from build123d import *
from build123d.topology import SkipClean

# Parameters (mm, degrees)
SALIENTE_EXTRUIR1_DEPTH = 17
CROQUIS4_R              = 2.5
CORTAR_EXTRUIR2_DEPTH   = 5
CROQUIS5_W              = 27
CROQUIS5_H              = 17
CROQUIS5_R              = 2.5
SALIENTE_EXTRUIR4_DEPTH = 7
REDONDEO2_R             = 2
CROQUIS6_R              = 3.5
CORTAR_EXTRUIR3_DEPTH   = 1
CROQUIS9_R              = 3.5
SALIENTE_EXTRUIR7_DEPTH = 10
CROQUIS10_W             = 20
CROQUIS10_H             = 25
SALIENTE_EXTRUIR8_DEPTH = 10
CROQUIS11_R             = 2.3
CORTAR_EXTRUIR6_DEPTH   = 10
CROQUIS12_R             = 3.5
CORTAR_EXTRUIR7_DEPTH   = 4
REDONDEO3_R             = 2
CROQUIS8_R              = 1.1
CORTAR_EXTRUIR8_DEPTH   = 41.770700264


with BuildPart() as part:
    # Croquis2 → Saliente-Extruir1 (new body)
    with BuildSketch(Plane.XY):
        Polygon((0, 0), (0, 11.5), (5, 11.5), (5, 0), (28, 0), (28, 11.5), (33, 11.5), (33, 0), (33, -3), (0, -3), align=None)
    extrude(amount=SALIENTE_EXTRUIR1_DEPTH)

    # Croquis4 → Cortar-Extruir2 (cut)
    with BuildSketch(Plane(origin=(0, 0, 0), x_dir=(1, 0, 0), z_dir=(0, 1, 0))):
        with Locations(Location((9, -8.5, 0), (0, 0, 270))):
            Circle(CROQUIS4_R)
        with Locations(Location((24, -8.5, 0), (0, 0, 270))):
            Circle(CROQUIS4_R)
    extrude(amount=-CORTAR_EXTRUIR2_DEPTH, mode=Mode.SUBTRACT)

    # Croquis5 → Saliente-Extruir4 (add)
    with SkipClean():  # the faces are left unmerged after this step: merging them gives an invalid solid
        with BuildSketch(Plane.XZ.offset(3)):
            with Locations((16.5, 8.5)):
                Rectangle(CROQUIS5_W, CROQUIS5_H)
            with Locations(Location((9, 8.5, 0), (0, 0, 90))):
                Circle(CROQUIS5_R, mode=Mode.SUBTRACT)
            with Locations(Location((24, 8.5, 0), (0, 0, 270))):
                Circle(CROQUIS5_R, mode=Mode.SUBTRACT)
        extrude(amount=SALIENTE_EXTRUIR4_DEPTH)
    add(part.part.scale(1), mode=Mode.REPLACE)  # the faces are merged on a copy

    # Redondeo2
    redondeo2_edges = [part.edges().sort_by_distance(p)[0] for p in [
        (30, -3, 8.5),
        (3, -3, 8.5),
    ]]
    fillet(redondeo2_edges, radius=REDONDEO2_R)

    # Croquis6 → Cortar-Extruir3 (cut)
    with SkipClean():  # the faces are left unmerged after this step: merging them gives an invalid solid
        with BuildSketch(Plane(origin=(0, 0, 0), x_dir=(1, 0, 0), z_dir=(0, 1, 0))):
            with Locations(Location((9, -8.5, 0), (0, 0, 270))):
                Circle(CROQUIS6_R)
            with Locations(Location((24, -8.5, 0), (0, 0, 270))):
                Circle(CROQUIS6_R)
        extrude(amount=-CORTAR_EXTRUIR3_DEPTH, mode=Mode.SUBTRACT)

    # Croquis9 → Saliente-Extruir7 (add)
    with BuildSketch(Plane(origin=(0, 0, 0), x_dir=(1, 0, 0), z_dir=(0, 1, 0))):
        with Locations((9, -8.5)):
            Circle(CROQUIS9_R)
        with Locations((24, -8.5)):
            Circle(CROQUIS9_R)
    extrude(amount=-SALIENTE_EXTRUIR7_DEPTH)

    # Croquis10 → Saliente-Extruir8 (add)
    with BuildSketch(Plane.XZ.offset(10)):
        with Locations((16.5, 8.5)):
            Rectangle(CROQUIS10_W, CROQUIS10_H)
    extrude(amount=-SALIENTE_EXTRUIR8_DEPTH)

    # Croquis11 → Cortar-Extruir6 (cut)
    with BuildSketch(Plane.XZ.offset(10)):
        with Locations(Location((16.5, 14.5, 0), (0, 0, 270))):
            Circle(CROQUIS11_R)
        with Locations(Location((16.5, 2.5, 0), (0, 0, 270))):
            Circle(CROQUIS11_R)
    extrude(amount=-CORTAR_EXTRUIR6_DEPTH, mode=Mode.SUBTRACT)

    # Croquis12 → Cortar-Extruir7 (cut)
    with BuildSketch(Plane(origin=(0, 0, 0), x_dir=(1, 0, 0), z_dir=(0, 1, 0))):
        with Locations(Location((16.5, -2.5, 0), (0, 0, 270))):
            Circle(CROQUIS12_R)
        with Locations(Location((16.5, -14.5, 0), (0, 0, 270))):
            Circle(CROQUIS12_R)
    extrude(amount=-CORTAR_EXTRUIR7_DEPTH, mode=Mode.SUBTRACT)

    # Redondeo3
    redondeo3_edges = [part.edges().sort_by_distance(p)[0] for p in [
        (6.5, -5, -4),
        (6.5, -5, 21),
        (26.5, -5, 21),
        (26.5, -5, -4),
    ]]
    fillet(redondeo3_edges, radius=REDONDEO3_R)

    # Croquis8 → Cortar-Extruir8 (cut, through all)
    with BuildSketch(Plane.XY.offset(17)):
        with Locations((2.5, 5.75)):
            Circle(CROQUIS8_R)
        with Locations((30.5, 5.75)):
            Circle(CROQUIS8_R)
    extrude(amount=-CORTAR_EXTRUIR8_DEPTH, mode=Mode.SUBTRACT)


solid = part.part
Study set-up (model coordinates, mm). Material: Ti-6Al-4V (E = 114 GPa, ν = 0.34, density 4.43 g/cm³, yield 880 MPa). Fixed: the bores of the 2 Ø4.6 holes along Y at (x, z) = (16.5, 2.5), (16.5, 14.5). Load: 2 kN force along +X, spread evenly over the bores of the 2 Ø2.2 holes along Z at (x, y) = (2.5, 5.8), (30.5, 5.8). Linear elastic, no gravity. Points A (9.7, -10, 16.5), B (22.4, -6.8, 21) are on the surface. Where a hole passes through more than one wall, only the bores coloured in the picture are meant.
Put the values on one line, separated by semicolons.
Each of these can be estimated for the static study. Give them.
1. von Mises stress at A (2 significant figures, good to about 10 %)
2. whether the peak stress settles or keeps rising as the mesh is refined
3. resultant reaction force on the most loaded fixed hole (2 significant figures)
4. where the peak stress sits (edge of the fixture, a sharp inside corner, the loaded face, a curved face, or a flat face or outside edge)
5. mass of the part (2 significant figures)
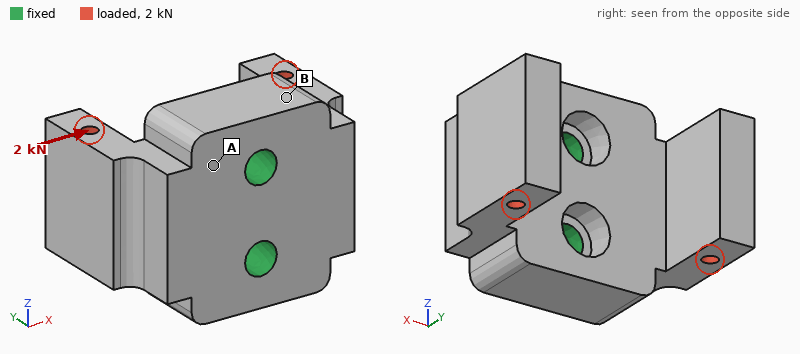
30 MPa; keeps rising; 1.0 kN; edge of the fixture; 35 g
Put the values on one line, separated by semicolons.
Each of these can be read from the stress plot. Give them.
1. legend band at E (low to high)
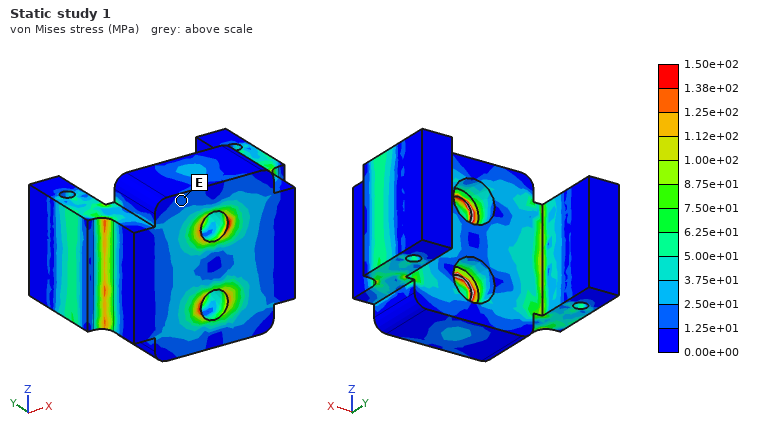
1.25e+01 to 2.50e+01 MPa
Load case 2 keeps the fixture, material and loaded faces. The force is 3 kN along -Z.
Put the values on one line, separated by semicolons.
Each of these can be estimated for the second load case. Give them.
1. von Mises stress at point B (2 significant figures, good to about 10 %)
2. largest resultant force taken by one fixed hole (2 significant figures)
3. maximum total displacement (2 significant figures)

23 MPa; 2.7 kN; 30 µm
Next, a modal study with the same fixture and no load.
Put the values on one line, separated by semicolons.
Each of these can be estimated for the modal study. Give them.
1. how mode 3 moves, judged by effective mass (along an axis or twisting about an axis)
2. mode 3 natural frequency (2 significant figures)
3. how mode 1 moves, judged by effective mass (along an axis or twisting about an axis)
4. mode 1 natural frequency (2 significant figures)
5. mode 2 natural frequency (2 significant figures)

along Z; 19 kHz; along X; 10 kHz; 13 kHz
